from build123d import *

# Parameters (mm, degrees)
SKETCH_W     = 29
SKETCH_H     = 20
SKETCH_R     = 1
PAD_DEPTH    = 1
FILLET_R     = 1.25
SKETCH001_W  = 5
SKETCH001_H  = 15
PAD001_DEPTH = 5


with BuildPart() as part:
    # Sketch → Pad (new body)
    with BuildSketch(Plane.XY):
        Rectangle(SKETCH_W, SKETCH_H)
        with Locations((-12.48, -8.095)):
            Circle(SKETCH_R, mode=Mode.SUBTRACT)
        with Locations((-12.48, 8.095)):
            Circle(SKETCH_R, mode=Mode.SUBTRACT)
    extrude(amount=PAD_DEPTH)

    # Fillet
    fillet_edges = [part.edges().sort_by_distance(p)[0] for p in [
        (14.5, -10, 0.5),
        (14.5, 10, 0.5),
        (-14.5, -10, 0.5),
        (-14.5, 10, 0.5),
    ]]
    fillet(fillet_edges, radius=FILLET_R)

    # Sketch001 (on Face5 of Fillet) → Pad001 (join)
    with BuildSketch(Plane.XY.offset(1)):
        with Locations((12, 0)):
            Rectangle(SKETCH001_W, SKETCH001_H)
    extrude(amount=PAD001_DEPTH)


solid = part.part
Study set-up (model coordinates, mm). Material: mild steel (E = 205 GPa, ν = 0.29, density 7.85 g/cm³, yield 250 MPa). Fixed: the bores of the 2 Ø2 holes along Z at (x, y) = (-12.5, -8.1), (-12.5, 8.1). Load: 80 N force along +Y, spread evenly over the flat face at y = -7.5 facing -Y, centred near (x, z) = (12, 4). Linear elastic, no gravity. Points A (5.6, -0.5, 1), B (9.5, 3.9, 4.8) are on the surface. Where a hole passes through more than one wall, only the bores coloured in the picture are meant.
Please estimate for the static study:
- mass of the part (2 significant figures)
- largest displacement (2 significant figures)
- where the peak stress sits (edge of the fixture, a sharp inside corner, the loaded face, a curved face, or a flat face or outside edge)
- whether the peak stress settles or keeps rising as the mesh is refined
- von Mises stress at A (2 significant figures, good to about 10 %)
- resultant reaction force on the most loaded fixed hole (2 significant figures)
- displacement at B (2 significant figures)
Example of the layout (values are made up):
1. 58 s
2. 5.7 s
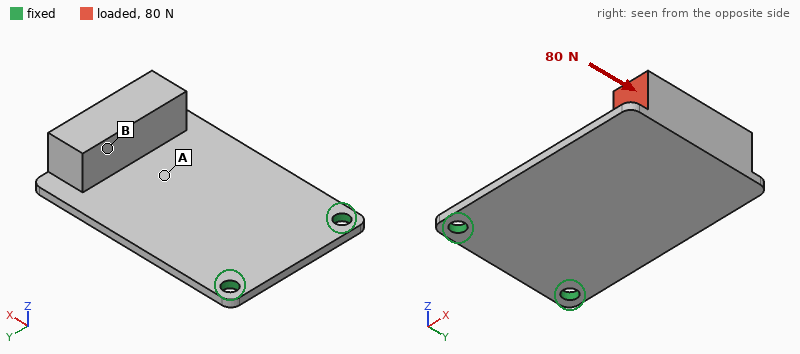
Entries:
1. 7.4 g
2. 62 µm
3. edge of the fixture
4. keeps rising
5. 50 MPa
6. 130 N
7. 38 µm
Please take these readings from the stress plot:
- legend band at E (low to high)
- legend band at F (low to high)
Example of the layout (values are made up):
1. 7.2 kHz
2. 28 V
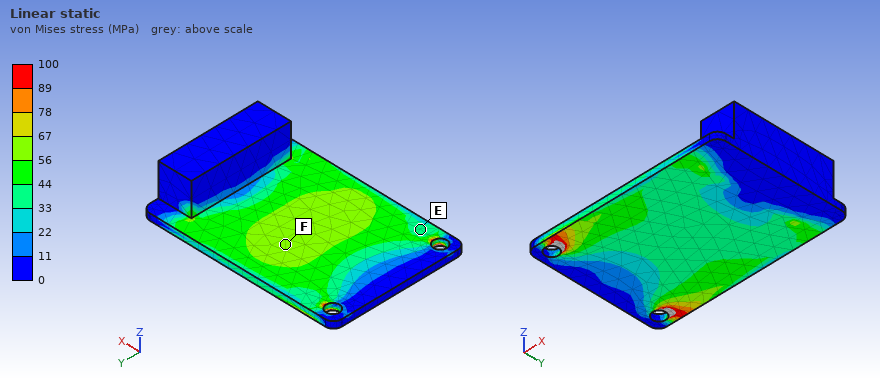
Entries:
1. 33 to 44 MPa
2. 56 to 67 MPa
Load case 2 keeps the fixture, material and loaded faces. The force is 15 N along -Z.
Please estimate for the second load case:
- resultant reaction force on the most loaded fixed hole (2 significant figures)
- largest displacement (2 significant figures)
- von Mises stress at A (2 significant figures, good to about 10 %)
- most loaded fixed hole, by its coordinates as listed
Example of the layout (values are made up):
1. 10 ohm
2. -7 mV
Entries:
1. 14 N
2. 0.29 mm
3. 34 MPa
4. (-12.5, -8.1)
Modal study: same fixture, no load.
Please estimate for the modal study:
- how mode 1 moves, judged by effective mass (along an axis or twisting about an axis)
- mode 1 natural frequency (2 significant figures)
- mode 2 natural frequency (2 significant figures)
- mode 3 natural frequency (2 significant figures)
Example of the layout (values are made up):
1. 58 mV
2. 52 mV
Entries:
1. along Z
2. 610 Hz
3. 2500 Hz
4. 4800 Hz
